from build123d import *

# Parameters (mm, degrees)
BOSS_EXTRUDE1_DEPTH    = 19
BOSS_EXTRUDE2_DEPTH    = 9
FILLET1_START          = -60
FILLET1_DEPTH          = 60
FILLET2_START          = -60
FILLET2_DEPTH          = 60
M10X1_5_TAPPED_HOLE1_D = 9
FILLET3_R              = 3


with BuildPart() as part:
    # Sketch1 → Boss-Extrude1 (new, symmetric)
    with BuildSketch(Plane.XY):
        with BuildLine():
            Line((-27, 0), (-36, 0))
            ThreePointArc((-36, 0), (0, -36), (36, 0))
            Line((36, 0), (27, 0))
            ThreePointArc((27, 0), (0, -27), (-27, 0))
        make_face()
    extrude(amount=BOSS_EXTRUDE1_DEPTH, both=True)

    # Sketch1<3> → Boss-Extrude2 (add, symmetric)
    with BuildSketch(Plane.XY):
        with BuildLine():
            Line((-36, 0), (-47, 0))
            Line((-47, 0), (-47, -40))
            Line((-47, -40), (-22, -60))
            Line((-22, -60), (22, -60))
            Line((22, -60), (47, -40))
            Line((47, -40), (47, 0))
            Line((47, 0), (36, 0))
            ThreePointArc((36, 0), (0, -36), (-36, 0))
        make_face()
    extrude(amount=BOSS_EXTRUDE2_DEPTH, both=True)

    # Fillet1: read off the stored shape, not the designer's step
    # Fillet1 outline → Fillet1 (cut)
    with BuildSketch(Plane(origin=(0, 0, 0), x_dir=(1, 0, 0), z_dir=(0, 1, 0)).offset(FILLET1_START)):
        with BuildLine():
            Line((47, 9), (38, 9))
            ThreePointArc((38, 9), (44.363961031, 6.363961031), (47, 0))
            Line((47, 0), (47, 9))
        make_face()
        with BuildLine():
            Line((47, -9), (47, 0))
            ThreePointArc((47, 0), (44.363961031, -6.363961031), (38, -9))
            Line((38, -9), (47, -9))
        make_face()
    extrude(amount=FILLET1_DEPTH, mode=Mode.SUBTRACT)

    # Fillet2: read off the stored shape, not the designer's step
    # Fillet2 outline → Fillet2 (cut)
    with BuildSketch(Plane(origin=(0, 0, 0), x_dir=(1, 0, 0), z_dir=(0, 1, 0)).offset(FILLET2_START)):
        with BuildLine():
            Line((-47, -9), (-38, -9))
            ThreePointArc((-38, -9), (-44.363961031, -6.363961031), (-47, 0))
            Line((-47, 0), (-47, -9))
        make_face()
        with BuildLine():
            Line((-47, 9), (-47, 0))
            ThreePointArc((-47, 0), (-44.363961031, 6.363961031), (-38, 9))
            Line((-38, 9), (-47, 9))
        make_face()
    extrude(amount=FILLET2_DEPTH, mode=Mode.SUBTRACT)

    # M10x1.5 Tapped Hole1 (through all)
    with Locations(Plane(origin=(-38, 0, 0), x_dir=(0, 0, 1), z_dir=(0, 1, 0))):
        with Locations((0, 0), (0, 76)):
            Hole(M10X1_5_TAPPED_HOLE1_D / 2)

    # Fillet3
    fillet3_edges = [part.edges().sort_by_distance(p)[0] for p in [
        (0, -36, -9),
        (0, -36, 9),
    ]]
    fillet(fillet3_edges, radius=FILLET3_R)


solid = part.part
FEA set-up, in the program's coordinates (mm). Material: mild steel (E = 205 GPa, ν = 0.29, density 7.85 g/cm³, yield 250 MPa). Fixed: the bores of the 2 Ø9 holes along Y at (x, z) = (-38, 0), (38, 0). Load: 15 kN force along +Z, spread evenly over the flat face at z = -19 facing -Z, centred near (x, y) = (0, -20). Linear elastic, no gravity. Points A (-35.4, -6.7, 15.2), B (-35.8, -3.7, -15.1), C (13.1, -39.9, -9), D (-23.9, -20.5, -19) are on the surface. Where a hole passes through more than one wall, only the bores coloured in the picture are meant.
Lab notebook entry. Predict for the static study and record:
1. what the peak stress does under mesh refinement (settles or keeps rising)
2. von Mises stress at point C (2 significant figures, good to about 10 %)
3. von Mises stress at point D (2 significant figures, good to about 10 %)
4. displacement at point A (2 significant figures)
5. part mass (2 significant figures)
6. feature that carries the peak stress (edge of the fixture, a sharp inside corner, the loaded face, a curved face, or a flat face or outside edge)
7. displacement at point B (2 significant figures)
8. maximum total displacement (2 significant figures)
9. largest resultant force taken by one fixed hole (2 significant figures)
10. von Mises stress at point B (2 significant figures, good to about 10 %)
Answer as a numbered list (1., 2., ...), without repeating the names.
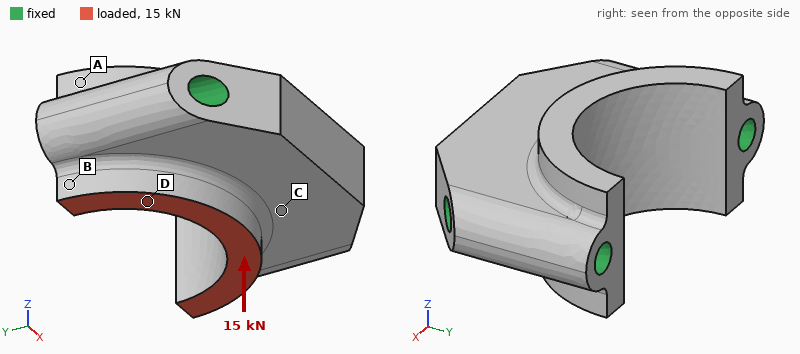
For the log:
1. keeps rising
2. 8.9 MPa
3. 15 MPa
4. 1.3 µm
5. 640 g
6. edge of the fixture
7. 2.0 µm
8. 5.2 µm
9. 7.5 kN
10. 18 MPa
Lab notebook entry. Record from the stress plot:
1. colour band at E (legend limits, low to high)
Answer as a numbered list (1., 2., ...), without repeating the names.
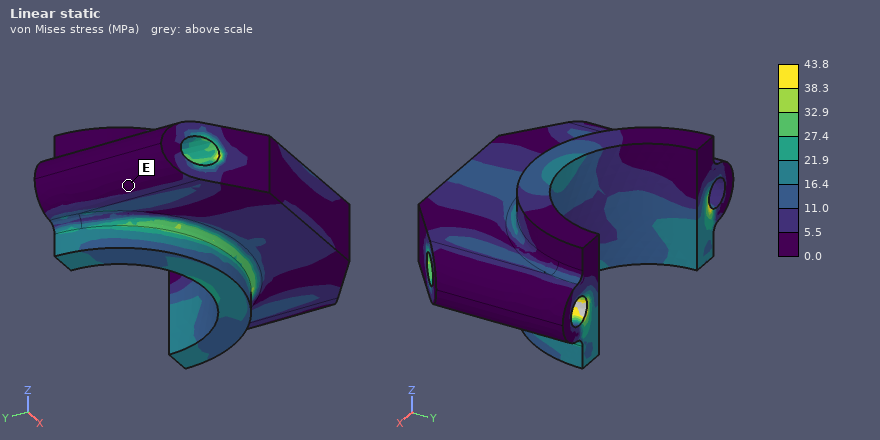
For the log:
1. 0.0 to 5.5 MPa
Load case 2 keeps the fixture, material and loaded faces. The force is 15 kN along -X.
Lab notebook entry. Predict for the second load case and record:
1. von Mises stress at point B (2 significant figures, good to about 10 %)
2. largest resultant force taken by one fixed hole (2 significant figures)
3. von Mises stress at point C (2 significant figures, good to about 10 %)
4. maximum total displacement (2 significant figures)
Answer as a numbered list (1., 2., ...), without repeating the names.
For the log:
1. 42 MPa
2. 8.1 kN
3. 9.6 MPa
4. 13 µm
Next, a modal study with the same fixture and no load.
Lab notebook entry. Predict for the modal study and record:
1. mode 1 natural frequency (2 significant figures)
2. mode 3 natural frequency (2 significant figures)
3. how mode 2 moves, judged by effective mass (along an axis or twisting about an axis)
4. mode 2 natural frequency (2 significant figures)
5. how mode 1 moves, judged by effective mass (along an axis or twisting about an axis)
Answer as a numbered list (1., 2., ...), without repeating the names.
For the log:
1. 12 kHz
2. 20 kHz
3. along Y
4. 19 kHz
5. along Z
